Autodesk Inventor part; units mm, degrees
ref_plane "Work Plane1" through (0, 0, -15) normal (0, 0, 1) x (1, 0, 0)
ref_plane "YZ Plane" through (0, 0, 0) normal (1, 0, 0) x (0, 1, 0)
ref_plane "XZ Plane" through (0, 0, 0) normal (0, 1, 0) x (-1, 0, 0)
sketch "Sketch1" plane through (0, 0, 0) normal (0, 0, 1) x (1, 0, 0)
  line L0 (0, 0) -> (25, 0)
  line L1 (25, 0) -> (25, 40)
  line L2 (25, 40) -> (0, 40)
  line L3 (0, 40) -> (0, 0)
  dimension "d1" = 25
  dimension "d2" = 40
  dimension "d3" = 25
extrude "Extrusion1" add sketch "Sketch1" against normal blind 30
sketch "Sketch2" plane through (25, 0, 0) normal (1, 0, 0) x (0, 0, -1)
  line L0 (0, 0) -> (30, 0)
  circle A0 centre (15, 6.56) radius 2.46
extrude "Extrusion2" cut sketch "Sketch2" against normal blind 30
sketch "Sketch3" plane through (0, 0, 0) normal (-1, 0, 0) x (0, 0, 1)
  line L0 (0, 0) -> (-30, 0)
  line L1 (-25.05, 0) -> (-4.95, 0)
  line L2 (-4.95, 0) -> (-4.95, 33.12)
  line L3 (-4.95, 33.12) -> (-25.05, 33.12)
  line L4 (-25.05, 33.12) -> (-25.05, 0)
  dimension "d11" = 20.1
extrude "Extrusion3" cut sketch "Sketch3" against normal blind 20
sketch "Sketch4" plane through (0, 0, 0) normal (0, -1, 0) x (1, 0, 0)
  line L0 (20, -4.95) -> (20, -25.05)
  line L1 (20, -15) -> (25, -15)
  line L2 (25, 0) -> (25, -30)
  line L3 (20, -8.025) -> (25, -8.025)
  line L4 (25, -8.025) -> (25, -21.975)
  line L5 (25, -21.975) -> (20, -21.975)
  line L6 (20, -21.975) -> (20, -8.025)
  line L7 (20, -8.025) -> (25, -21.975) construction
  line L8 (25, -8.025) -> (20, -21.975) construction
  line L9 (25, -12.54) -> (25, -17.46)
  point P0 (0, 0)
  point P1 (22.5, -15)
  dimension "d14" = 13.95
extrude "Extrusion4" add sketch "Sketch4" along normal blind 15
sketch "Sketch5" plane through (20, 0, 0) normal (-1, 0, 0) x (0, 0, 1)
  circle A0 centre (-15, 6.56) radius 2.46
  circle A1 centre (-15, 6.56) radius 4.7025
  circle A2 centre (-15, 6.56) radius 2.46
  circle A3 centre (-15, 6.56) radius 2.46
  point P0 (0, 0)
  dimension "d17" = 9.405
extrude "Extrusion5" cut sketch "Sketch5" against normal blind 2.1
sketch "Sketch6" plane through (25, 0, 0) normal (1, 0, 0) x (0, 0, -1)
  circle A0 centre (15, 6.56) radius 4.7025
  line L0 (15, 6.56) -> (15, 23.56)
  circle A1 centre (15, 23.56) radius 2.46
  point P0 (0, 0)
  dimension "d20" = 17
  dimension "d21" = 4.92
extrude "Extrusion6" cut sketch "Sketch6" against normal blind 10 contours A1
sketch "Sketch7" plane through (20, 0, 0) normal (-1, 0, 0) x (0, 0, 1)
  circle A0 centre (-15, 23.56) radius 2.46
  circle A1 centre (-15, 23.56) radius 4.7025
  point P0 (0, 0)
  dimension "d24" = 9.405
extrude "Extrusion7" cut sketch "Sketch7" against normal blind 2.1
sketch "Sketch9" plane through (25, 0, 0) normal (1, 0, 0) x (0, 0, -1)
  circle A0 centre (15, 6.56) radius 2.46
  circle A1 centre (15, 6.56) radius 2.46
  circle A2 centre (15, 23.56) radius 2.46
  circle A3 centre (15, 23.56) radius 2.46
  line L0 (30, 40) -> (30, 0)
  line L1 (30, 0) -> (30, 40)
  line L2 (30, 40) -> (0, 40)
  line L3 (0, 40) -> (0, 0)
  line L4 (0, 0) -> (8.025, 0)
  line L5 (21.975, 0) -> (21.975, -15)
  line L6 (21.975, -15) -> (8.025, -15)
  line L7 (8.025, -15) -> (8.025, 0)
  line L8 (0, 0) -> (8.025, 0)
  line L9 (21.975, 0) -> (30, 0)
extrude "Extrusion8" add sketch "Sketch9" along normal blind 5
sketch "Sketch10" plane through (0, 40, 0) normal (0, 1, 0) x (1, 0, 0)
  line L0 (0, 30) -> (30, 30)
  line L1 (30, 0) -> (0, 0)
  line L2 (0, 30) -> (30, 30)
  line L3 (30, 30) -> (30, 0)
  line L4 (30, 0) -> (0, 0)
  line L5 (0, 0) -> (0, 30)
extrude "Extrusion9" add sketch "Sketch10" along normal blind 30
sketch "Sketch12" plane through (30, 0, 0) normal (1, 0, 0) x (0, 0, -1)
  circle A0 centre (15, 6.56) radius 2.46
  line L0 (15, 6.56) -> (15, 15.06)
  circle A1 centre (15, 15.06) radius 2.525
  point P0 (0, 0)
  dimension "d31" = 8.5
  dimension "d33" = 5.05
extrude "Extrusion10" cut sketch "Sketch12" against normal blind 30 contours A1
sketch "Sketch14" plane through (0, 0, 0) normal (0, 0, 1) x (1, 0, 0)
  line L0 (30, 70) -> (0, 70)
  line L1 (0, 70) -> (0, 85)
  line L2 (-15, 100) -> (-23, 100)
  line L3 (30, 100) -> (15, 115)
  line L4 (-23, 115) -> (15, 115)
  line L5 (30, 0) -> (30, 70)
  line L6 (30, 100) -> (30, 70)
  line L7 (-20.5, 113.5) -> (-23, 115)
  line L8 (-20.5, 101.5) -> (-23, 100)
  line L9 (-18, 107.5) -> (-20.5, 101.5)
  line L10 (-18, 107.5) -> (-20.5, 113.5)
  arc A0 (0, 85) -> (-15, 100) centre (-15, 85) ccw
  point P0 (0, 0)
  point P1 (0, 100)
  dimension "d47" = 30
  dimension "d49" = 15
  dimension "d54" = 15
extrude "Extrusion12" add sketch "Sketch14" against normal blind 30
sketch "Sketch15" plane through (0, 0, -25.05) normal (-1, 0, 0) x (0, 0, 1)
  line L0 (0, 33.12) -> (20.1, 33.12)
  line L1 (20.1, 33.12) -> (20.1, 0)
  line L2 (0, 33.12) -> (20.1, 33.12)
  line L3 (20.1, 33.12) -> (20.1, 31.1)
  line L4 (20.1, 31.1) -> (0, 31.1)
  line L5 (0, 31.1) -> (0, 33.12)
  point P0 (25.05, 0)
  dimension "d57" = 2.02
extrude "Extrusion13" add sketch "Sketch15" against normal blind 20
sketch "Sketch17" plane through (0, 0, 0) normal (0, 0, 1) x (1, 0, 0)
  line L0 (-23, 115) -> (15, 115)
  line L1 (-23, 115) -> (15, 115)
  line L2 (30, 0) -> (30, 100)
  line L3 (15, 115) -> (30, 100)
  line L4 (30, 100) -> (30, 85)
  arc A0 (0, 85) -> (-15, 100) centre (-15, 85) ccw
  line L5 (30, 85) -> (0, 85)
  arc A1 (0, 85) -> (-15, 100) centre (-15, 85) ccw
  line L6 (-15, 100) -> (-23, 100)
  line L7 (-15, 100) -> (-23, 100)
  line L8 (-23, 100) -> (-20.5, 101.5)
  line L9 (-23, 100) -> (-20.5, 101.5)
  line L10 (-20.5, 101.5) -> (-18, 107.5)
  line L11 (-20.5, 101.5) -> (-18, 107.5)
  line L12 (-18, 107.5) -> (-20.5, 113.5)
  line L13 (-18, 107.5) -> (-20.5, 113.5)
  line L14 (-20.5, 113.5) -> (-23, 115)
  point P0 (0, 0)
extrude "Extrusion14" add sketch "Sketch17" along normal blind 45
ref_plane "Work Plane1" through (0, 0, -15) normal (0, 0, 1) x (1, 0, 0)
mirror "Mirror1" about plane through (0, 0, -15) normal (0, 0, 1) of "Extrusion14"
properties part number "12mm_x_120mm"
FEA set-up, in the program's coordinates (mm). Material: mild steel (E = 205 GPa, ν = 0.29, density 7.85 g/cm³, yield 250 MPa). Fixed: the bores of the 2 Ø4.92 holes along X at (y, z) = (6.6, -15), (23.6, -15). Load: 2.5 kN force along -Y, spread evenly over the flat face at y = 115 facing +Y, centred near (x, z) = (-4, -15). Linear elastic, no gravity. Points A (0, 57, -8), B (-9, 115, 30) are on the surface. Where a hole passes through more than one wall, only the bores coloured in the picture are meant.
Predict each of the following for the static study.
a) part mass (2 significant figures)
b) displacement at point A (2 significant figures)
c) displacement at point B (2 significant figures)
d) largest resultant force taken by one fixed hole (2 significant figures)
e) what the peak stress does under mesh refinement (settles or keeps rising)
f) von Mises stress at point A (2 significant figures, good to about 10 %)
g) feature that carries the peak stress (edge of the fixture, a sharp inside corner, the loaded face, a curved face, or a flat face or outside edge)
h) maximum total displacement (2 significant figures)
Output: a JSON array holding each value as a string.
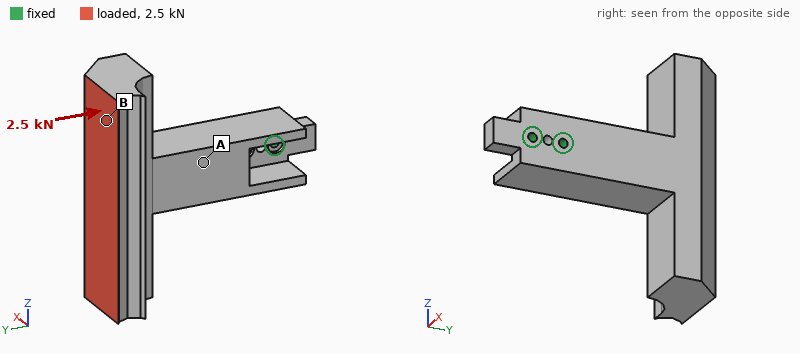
["1.6 kg", "25 µm", "67 µm", "3.4 kN", "keeps rising", "13 MPa", "edge of the fixture", "73 µm"]
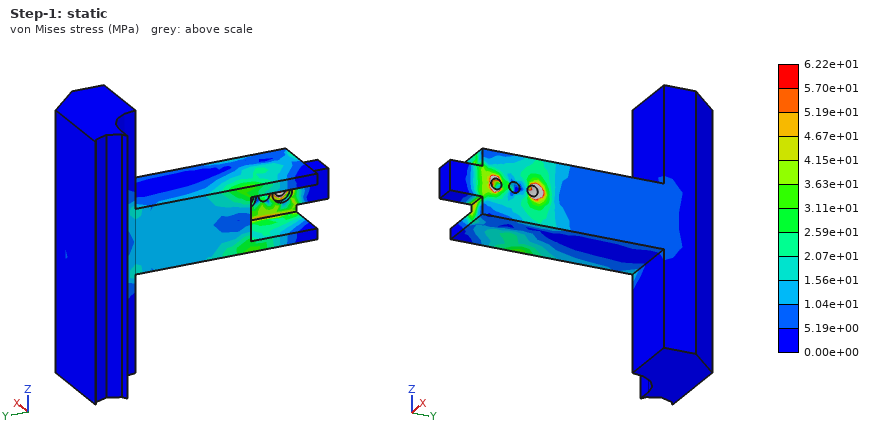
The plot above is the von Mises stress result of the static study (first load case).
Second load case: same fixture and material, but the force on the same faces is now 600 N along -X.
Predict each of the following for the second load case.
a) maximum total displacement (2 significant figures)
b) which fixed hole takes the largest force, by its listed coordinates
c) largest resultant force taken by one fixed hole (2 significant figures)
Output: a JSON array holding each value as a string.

["53 µm", "(23.6, -15)", "2.8 kN"]
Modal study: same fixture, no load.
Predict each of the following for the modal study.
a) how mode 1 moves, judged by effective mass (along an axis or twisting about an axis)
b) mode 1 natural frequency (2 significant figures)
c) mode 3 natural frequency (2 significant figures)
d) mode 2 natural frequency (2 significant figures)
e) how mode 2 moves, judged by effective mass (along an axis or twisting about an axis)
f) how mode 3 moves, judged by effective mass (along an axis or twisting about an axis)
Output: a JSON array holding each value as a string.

["along X", "610 Hz", "880 Hz", "650 Hz", "along Z", "twisting about Y"]
